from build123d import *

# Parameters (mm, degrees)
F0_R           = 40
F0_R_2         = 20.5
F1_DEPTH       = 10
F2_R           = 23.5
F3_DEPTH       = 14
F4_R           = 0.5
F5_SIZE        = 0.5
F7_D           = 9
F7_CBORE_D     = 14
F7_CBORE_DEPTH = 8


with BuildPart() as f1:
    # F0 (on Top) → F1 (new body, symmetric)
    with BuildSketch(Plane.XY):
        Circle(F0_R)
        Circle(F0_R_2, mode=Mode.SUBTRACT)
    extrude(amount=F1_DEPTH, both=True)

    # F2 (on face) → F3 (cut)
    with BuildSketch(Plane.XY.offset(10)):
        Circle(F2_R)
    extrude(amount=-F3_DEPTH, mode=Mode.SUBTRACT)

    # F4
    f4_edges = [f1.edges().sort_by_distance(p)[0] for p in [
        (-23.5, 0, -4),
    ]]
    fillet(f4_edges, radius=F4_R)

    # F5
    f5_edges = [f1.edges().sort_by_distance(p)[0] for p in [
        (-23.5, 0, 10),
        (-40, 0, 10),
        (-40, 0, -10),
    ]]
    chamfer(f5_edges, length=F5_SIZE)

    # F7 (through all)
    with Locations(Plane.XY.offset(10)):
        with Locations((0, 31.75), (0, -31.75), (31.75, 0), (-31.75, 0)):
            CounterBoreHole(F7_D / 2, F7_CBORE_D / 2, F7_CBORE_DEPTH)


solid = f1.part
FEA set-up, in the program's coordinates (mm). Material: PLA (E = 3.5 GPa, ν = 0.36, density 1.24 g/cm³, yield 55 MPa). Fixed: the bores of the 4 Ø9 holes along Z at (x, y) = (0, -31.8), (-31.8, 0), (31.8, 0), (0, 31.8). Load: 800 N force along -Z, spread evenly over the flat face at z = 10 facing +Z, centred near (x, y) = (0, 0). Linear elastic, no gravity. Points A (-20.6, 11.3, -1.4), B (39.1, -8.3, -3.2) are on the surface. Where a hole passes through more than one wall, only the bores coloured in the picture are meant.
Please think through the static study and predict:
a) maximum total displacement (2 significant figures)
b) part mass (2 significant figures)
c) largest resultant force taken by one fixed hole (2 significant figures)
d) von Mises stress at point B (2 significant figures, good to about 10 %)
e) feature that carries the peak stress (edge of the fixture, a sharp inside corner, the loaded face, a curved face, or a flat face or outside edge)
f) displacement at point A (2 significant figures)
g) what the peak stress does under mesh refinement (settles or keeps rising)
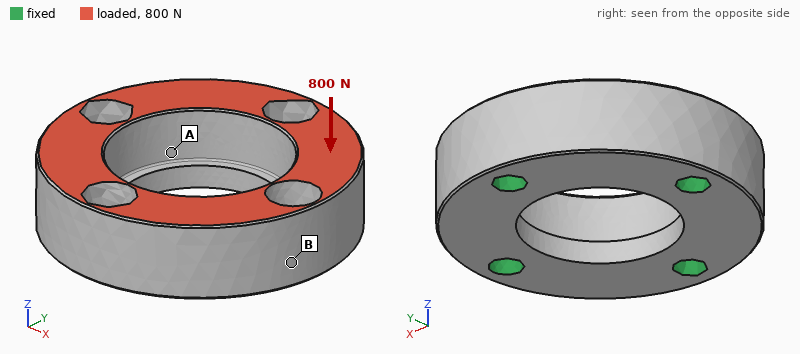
11 µm
75 g
210 N
0.80 MPa
edge of the fixture
3.5 µm
keeps rising
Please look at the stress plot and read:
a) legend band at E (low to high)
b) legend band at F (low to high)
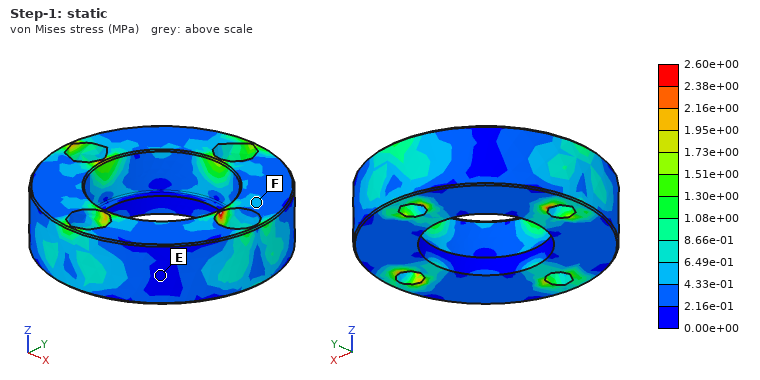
0.00e+00 to 2.16e-01 MPa
4.33e-01 to 6.49e-01 MPa
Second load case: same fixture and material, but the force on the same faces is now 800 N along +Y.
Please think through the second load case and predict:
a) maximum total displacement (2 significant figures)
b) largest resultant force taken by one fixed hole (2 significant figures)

19 µm
270 N
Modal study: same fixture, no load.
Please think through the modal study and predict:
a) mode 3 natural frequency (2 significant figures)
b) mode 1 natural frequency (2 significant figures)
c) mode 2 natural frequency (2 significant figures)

5900 Hz
5400 Hz
5900 Hz
